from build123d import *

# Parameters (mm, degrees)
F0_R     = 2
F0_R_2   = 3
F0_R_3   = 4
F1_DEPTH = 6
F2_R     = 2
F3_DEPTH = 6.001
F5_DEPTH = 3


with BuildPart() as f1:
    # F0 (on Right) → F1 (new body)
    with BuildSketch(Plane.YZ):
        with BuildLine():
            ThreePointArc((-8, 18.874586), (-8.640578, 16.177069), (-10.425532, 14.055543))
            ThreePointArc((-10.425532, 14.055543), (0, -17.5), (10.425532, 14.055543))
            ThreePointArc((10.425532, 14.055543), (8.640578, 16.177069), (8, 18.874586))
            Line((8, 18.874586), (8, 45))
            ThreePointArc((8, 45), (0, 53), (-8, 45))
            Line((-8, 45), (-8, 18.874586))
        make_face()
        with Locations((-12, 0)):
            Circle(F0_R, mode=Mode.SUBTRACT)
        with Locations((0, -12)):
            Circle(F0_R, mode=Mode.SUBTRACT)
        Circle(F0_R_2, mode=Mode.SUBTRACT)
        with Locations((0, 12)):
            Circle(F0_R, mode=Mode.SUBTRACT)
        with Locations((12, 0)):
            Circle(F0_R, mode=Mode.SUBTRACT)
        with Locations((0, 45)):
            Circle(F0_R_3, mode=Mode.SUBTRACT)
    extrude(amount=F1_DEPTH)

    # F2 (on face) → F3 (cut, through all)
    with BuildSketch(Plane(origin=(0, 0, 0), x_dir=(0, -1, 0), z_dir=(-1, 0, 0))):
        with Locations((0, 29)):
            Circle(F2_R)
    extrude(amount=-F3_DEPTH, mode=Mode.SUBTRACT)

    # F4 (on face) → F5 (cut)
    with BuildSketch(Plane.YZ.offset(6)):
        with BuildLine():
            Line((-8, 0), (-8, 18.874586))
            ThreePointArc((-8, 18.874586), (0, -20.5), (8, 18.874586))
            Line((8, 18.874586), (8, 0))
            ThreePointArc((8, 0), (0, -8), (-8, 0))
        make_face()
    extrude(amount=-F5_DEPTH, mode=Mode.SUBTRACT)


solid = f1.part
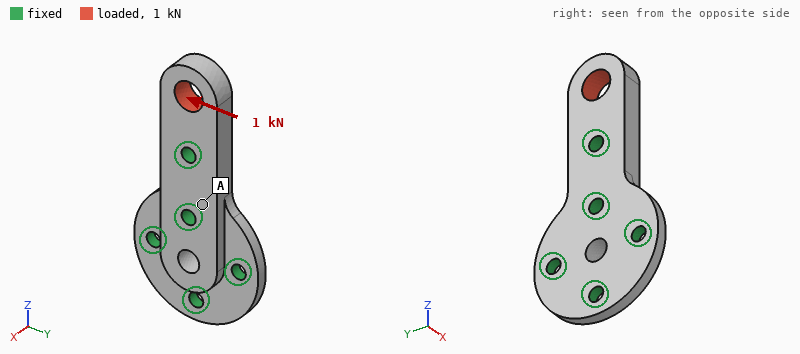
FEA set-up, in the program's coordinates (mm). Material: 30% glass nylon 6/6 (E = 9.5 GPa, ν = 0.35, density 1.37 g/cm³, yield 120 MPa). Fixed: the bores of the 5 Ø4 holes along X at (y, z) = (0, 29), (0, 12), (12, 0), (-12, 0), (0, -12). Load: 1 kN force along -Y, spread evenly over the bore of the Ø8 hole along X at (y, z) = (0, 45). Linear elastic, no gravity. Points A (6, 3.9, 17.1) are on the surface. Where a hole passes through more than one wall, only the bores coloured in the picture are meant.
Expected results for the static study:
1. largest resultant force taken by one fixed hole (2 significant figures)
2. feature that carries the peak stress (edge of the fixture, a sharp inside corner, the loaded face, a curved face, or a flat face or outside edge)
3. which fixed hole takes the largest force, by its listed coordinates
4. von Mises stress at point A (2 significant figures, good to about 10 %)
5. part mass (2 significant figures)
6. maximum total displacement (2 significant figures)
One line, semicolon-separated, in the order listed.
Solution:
1.5 kN; edge of the fixture; (0, 29); 15 MPa; 9.0 g; 0.35 mm
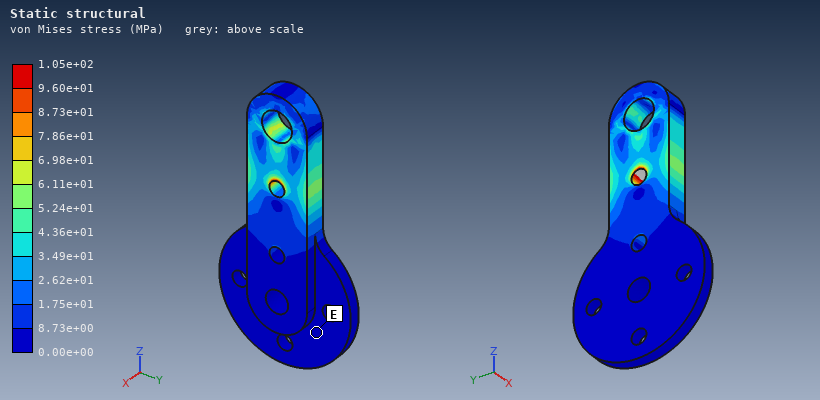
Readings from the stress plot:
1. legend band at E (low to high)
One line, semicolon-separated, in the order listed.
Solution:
0.00e+00 to 8.73e+00 MPa
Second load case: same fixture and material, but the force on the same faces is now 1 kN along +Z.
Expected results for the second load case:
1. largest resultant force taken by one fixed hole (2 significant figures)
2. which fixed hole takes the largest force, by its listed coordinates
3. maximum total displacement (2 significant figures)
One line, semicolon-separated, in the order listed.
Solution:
850 N; (0, 29); 41 µm
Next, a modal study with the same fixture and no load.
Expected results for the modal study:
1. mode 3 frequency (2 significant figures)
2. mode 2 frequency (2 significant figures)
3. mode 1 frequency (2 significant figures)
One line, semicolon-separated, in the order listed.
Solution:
12 kHz; 8300 Hz; 5300 Hz
